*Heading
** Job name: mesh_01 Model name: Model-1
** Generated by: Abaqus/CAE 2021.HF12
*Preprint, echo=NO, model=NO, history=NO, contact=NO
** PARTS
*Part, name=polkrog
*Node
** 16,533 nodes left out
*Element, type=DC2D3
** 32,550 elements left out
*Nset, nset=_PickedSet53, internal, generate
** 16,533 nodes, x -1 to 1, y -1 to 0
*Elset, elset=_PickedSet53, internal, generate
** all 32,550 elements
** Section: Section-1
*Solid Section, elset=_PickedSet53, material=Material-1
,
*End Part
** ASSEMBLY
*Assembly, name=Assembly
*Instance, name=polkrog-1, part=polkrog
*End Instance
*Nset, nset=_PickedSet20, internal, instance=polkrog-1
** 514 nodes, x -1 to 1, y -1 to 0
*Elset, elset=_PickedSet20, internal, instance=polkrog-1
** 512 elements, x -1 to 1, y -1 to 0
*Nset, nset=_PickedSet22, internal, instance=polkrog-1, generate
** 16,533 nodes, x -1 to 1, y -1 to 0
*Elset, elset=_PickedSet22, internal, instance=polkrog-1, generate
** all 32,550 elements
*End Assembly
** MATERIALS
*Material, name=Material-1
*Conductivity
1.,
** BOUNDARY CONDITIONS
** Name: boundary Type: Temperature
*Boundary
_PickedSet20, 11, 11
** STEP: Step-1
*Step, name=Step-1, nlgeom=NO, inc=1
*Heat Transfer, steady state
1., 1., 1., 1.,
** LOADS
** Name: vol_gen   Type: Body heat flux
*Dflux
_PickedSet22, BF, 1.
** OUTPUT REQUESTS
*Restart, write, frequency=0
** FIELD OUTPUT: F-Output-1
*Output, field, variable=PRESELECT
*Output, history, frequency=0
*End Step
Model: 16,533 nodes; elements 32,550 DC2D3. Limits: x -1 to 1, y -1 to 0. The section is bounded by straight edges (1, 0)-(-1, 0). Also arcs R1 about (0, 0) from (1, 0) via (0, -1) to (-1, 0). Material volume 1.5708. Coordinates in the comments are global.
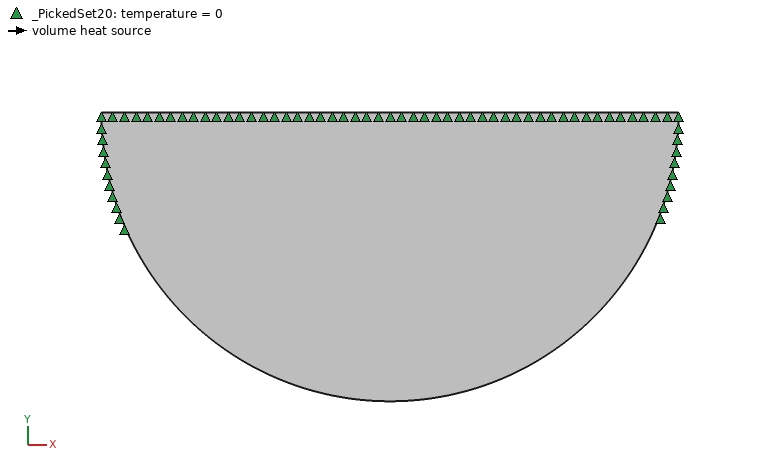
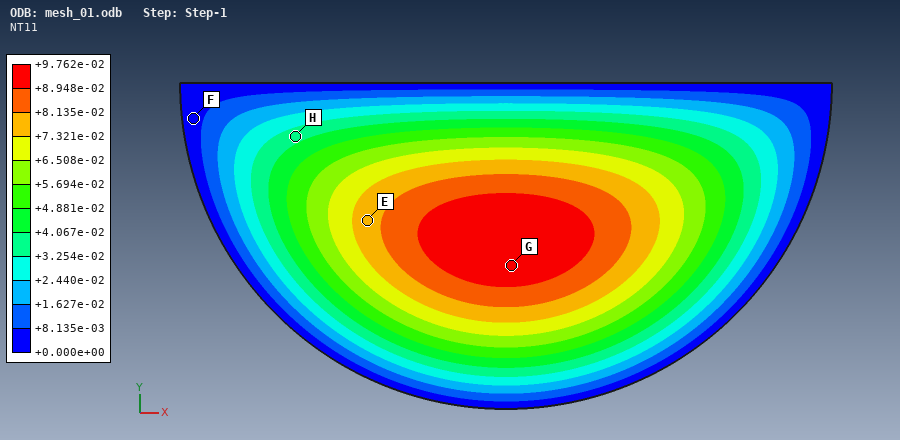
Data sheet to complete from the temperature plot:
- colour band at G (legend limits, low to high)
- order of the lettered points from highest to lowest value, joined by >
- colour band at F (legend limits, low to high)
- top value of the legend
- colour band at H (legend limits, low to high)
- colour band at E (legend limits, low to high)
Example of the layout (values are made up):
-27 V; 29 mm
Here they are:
+8.948e-02 to +9.762e-02; G > E > H > F; +0.000e+00 to +8.135e-03; +9.762e-02; +3.254e-02 to +4.067e-02; +7.321e-02 to +8.135e-02
